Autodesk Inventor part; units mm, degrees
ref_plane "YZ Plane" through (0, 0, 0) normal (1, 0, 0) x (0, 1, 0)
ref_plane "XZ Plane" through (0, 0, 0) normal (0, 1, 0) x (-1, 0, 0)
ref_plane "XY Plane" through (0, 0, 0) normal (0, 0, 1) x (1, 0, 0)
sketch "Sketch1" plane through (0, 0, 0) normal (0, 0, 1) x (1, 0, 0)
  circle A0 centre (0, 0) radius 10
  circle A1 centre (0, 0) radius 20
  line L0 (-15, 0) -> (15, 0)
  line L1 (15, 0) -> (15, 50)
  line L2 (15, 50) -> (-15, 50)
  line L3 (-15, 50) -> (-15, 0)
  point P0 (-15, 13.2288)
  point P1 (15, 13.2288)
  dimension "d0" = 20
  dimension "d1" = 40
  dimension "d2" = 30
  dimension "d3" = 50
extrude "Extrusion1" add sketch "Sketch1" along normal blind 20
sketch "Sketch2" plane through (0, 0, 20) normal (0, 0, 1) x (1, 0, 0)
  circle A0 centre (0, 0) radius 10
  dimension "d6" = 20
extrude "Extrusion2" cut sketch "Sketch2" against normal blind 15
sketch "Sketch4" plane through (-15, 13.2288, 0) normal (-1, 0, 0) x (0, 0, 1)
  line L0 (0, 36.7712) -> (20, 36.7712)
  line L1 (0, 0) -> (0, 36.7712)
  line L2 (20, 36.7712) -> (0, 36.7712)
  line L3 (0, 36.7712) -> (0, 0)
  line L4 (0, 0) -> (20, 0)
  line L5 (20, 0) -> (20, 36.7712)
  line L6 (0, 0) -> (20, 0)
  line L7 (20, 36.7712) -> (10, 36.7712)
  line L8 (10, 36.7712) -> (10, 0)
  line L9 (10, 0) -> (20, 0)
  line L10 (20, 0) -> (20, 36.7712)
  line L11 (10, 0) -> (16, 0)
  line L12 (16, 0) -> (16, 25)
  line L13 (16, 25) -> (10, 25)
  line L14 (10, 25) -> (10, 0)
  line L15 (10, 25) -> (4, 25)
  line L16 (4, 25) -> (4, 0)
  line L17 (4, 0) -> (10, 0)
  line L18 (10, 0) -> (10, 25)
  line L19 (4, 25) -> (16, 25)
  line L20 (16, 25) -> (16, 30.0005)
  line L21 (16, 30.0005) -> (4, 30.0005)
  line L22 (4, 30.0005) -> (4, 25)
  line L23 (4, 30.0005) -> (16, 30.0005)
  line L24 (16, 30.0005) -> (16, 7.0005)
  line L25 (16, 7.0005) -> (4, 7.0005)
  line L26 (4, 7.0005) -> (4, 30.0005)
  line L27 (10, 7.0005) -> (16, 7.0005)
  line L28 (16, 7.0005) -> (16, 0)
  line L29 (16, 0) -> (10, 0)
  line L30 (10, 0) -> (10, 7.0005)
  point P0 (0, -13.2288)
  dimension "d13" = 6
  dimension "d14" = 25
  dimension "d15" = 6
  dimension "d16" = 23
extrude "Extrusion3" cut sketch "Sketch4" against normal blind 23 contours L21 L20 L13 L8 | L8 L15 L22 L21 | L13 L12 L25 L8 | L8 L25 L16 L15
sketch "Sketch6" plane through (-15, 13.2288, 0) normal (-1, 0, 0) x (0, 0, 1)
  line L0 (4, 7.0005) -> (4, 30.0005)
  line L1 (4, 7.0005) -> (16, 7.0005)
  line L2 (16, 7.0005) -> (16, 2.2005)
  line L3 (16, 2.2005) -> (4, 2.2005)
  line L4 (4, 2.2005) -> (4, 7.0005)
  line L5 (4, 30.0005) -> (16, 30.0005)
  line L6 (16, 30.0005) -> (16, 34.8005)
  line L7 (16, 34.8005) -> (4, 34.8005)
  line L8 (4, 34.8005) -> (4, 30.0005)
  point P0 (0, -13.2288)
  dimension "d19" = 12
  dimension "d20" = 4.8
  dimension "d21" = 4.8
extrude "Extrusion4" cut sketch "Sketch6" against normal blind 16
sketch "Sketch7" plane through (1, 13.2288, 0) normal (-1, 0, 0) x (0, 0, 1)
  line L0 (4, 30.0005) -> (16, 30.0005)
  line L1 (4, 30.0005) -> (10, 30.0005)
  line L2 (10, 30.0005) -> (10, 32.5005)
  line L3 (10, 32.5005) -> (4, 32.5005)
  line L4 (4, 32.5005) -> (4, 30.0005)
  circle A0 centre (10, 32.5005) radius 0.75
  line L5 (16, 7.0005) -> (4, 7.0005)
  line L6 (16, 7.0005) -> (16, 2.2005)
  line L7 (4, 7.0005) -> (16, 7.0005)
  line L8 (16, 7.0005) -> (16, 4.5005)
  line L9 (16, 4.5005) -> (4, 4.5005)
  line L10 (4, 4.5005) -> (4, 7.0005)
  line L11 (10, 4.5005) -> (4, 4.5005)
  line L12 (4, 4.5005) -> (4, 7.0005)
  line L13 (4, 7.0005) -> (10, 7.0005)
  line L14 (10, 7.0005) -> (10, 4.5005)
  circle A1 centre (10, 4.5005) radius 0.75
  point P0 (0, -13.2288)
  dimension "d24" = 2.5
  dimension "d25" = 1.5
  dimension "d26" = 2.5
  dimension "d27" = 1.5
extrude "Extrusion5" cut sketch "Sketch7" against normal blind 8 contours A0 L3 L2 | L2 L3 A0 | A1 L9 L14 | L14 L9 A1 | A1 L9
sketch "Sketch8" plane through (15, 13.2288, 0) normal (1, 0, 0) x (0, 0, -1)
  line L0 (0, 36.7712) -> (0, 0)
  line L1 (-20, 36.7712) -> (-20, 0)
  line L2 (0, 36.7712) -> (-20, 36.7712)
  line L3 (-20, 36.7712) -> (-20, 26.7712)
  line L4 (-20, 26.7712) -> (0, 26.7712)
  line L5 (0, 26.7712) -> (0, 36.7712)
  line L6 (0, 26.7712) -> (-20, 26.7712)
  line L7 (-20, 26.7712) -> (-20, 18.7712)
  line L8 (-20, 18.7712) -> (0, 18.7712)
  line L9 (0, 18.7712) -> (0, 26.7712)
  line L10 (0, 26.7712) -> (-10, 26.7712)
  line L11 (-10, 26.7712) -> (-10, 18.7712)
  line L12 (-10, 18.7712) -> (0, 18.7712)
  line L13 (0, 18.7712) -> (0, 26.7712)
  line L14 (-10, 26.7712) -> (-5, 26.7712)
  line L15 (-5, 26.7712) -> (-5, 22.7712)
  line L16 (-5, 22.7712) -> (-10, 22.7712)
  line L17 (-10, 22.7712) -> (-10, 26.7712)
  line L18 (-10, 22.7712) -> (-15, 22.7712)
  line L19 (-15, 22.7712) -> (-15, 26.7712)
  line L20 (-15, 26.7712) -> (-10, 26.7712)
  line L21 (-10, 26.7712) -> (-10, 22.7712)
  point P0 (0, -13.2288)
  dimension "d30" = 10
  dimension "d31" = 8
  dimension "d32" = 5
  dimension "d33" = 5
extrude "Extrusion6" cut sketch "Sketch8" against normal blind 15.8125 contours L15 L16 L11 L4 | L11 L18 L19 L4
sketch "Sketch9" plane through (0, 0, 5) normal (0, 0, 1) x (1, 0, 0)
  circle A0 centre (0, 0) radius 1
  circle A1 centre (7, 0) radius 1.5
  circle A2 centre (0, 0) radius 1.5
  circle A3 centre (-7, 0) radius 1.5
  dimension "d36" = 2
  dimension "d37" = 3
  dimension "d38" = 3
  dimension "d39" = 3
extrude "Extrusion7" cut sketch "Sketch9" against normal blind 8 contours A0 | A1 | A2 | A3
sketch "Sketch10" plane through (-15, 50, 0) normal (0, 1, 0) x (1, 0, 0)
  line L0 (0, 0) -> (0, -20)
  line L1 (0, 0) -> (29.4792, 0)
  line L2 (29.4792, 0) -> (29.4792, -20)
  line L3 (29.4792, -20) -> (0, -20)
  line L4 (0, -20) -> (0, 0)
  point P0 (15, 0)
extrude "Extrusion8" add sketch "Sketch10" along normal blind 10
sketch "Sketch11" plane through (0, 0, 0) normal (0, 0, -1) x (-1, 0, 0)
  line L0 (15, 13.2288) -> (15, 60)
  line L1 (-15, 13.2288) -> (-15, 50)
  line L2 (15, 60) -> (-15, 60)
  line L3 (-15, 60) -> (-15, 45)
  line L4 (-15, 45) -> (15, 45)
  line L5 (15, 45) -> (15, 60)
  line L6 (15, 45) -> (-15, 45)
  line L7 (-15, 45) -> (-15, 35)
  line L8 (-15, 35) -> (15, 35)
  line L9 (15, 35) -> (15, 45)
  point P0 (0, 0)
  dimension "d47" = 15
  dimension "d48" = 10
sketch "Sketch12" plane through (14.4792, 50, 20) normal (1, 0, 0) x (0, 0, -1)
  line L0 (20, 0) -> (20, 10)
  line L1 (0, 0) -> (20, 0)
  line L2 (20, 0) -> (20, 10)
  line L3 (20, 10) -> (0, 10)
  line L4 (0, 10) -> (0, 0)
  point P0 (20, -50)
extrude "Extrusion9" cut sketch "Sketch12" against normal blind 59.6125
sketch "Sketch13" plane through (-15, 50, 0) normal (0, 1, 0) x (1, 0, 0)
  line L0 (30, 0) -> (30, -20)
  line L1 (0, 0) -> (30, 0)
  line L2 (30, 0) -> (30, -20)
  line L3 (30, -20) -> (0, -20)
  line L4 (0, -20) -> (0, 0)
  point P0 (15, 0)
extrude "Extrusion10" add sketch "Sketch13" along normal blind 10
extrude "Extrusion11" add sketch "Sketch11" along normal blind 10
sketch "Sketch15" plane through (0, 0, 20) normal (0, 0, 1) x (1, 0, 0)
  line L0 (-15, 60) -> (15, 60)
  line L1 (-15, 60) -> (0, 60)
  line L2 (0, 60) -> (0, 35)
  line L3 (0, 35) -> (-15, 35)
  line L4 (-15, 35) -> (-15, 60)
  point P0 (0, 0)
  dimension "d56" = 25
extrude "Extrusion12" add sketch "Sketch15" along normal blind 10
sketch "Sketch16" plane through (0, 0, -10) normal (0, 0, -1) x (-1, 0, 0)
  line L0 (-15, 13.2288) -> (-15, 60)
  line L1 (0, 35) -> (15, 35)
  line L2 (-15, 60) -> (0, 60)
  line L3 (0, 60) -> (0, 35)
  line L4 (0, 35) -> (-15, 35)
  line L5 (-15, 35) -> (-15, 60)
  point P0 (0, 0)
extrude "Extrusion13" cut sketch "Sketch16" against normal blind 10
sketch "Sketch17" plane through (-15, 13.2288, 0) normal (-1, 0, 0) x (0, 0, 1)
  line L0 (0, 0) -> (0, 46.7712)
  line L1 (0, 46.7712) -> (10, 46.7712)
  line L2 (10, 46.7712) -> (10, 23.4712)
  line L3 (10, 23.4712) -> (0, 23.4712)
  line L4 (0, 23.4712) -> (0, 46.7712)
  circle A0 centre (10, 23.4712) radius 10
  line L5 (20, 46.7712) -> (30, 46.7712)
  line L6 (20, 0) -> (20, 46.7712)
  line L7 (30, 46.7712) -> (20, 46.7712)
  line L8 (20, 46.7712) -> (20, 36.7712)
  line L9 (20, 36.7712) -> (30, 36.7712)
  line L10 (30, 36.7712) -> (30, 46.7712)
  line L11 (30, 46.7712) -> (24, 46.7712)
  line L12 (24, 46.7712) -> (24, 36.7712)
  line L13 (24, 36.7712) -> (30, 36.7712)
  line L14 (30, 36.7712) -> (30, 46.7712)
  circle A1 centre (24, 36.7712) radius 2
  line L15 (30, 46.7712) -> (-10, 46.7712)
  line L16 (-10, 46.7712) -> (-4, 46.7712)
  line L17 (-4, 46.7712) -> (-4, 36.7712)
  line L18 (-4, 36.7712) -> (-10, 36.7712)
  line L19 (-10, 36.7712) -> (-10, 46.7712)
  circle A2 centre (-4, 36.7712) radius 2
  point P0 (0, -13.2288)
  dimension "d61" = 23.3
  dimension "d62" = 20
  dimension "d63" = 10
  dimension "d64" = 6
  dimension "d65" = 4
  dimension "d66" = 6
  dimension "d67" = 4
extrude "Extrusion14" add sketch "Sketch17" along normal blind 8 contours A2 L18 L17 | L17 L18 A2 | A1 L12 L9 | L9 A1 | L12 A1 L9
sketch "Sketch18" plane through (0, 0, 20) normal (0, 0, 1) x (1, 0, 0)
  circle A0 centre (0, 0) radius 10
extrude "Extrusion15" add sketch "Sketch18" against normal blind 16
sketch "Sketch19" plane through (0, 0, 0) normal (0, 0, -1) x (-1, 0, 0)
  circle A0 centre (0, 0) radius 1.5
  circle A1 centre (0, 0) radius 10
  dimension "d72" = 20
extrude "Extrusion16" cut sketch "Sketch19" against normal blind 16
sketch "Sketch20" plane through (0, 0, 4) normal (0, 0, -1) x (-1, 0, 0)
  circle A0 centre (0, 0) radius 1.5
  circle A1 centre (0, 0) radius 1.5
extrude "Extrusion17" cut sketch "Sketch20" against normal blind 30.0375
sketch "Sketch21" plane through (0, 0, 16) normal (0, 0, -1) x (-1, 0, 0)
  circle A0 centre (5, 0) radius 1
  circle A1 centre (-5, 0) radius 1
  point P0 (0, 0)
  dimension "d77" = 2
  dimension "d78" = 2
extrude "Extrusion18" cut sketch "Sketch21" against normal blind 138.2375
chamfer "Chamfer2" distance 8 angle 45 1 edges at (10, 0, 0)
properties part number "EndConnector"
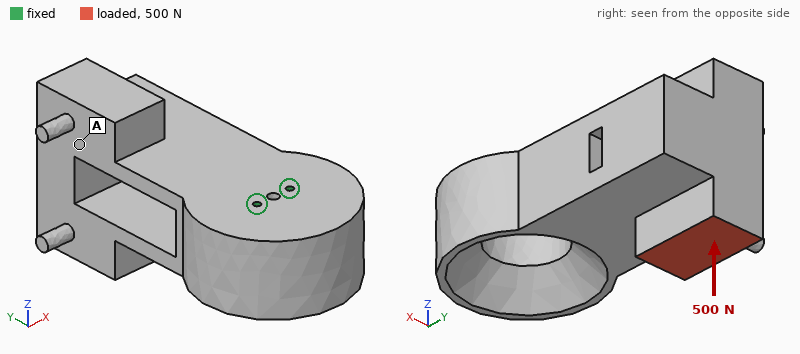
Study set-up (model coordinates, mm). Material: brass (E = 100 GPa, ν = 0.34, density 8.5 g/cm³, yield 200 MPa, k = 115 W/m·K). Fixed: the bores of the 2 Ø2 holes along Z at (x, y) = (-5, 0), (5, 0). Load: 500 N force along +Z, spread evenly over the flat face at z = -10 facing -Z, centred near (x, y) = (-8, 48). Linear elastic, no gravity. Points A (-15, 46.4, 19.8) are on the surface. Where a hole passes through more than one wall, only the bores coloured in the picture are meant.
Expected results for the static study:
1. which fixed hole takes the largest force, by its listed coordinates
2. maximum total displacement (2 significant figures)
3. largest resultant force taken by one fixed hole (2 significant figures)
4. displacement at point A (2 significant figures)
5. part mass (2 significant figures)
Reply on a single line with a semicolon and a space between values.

(-5, 0); 0.40 mm; 510 N; 0.29 mm; 360 g
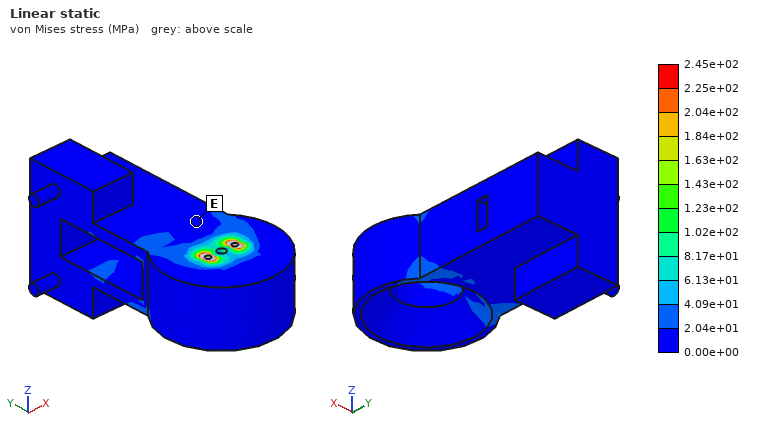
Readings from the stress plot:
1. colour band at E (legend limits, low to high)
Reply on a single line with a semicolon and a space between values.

0.00e+00 to 2.04e+01 MPa
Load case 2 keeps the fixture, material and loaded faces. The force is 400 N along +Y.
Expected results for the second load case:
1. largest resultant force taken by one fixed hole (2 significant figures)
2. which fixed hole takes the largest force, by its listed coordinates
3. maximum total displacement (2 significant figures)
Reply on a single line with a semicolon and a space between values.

470 N; (-5, 0); 0.18 mm
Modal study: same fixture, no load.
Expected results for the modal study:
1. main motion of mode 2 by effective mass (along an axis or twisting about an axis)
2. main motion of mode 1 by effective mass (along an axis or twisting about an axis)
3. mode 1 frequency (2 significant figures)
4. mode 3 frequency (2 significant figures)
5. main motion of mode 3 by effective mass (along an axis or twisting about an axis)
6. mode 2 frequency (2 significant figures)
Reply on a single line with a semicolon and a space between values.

along X; along Z; 460 Hz; 2100 Hz; twisting about Y; 1200 Hz
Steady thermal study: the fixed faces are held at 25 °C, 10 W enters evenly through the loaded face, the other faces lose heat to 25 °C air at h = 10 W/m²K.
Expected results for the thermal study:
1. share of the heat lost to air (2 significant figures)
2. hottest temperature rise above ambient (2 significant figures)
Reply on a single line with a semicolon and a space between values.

12 %; 18 K
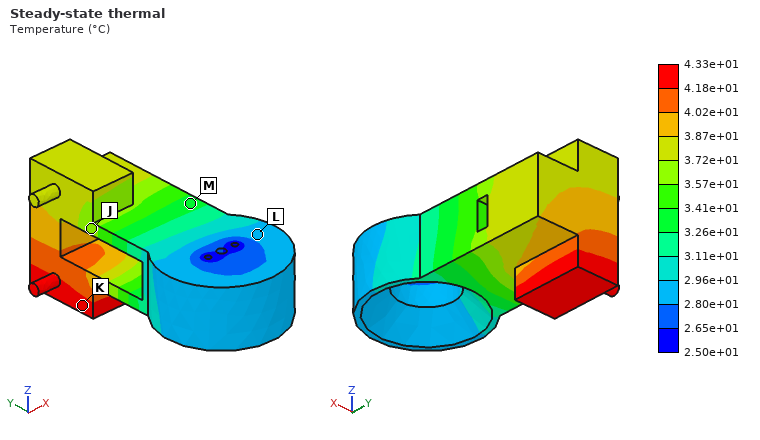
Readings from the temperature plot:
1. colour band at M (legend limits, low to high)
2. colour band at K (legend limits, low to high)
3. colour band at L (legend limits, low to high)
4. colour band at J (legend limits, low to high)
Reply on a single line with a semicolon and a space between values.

3.26e+01 to 3.41e+01 °C; 4.18e+01 to 4.33e+01 °C; 2.80e+01 to 2.96e+01 °C; 3.57e+01 to 3.72e+01 °C
